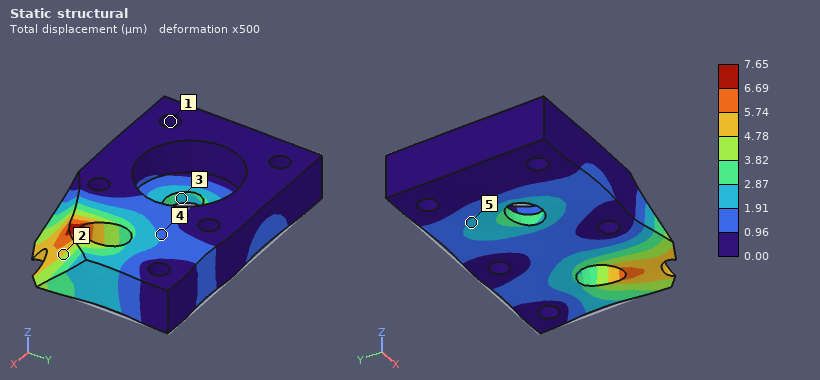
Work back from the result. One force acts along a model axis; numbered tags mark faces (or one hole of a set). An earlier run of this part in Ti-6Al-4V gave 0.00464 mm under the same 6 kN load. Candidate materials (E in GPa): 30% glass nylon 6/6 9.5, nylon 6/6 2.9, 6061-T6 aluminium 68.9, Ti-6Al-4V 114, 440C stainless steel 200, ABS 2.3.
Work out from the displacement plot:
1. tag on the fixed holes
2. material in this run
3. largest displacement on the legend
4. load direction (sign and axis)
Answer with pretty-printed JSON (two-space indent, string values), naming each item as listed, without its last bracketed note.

{
  "tag on the fixed holes": "1",
  "material in this run": "6061-T6 aluminium",
  "largest displacement on the legend": "7.65 µm",
  "load direction": "-Y"
}
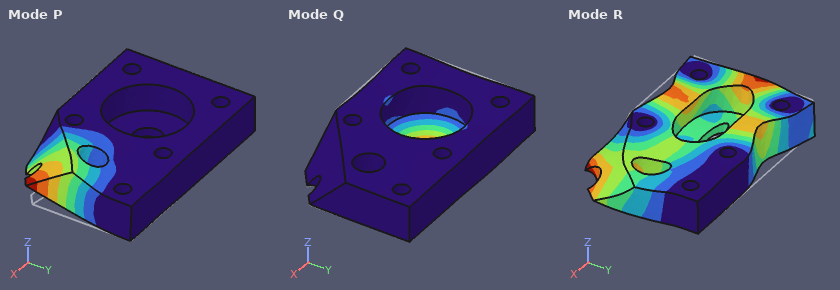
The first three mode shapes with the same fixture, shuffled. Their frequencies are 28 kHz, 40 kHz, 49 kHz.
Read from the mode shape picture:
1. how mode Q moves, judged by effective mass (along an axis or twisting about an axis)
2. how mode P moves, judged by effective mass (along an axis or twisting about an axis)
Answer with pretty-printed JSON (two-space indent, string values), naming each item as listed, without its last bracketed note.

{
  "how mode Q moves, judged by effective mass": "along Z",
  "how mode P moves, judged by effective mass": "along Z"
}
